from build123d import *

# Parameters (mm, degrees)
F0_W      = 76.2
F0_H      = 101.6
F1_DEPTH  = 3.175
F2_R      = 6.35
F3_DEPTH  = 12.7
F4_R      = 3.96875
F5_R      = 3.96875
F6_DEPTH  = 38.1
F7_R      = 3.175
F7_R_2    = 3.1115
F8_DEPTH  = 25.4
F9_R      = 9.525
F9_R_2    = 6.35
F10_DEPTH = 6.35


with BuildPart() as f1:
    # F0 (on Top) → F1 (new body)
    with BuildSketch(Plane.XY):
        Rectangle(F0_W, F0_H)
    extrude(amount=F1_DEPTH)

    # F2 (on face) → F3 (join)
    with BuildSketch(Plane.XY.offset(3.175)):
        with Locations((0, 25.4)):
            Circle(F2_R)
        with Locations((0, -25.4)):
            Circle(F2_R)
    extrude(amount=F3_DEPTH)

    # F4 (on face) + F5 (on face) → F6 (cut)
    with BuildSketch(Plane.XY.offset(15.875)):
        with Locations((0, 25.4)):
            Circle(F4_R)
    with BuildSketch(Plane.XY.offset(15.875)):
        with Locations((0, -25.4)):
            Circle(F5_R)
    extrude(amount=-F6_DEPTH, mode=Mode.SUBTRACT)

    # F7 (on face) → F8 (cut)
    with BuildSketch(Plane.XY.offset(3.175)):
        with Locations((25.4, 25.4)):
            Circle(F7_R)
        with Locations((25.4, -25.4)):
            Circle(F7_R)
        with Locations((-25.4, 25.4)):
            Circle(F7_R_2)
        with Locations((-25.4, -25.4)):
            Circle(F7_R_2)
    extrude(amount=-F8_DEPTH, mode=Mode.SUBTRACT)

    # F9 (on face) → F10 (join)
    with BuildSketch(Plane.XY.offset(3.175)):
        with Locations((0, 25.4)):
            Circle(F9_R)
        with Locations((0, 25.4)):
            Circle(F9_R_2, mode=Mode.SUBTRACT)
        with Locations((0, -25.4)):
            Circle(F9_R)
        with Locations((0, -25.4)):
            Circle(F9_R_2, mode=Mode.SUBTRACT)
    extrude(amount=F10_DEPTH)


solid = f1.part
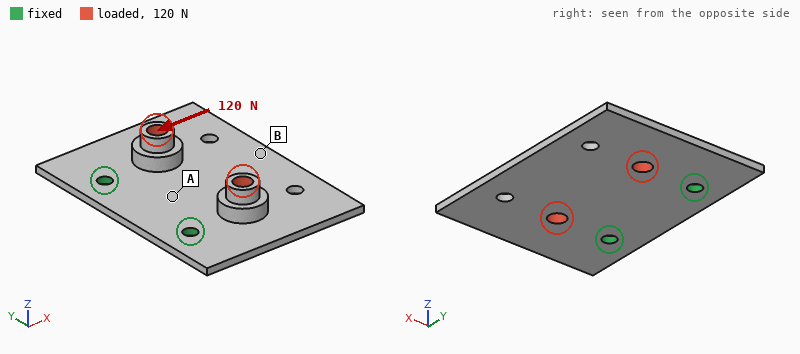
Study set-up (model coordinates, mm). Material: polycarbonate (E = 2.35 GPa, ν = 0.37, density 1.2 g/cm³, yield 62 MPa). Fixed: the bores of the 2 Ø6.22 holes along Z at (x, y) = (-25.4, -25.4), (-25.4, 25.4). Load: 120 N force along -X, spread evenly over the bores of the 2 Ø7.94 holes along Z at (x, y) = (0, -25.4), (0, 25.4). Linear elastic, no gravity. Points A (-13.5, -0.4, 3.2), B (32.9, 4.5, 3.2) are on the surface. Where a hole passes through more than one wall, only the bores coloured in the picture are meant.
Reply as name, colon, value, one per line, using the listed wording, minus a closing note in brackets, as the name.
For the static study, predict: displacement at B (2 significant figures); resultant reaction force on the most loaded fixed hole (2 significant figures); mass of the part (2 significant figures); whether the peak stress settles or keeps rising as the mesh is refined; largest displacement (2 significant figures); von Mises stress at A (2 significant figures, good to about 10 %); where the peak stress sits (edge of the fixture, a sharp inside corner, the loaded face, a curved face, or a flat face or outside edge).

displacement at B: 1.3 mm
resultant reaction force on the most loaded fixed hole: 60 N
mass of the part: 33 g
whether the peak stress settles or keeps rising as the mesh is refined: keeps rising
largest displacement: 1.4 mm
von Mises stress at A: 2.9 MPa
where the peak stress sits: edge of the fixture
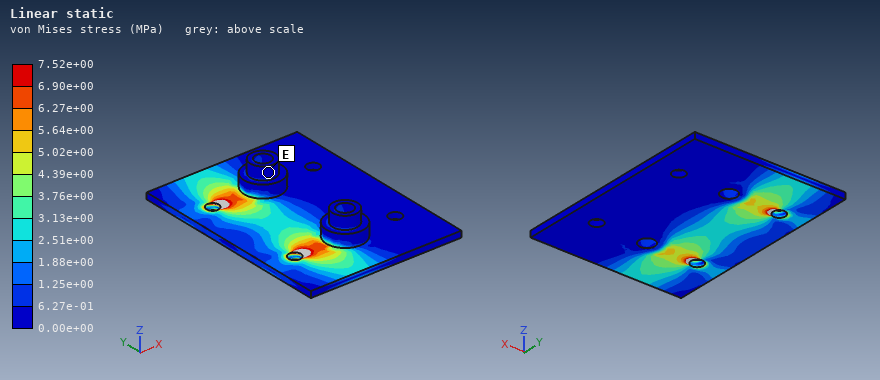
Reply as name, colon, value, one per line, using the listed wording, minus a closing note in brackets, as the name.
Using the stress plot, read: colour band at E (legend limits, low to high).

colour band at E: 0.00e+00 to 6.27e-01 MPa
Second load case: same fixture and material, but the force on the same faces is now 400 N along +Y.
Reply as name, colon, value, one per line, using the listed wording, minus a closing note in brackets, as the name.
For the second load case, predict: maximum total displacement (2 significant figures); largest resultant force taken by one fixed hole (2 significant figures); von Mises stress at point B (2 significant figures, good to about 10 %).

maximum total displacement: 1.5 mm
largest resultant force taken by one fixed hole: 270 N
von Mises stress at point B: 2.0 MPa
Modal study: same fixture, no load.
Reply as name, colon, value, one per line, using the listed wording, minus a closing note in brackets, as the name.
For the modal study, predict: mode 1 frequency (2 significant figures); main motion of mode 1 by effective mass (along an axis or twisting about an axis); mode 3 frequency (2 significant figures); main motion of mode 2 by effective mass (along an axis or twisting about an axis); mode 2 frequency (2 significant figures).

mode 1 frequency: 180 Hz
main motion of mode 1 by effective mass: along Z
mode 3 frequency: 660 Hz
main motion of mode 2 by effective mass: twisting about X
mode 2 frequency: 310 Hz
